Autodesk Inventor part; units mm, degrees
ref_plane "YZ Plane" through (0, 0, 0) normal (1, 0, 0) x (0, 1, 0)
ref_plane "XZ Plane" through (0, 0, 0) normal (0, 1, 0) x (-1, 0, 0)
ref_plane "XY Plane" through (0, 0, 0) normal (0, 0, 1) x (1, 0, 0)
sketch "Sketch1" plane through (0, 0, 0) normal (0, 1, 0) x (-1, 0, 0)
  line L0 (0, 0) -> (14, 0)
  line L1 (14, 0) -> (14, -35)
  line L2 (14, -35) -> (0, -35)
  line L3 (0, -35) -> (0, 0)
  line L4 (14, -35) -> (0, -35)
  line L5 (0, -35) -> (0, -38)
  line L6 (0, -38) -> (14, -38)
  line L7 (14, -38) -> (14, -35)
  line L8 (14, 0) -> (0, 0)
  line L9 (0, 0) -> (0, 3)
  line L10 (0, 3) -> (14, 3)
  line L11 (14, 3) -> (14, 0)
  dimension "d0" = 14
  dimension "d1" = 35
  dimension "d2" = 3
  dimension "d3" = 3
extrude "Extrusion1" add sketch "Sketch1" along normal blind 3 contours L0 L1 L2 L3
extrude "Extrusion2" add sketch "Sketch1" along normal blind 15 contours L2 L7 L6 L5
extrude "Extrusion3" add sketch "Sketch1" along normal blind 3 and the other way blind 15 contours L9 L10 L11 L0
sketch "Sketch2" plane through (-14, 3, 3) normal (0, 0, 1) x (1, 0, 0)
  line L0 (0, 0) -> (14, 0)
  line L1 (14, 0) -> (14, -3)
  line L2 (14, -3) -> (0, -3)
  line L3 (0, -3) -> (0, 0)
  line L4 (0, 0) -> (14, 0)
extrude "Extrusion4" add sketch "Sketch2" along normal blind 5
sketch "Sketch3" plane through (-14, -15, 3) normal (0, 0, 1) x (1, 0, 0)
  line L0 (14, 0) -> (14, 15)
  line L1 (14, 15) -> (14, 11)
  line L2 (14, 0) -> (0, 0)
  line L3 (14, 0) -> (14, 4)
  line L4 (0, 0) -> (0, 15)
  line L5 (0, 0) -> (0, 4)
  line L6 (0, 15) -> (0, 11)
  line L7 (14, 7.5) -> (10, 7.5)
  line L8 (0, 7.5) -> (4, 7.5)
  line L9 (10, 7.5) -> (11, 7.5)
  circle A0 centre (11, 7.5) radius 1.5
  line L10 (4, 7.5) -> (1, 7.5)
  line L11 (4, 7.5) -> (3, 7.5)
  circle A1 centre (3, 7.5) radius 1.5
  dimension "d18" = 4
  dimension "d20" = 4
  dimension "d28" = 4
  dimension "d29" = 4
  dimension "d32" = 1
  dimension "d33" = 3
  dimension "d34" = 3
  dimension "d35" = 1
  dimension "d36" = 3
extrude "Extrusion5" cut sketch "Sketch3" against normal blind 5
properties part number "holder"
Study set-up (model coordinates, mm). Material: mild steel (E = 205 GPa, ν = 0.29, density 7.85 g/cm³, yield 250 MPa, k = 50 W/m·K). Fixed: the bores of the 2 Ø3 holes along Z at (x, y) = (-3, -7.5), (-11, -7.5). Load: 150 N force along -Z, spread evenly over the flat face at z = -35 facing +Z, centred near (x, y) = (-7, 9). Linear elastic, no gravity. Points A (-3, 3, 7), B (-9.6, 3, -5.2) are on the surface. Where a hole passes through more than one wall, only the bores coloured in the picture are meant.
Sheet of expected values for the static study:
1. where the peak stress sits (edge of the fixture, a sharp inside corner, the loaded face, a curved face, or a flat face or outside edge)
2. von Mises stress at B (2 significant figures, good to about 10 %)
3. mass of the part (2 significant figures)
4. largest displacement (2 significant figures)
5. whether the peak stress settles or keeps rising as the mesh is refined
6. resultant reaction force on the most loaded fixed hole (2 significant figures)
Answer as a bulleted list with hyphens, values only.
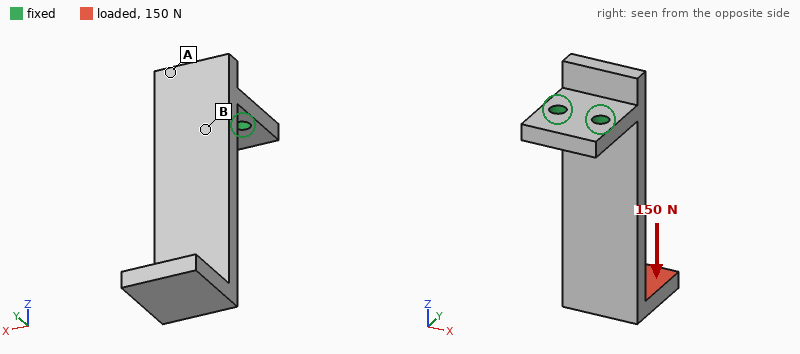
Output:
- edge of the fixture
- 55 MPa
- 24 g
- 0.25 mm
- keeps rising
- 76 N
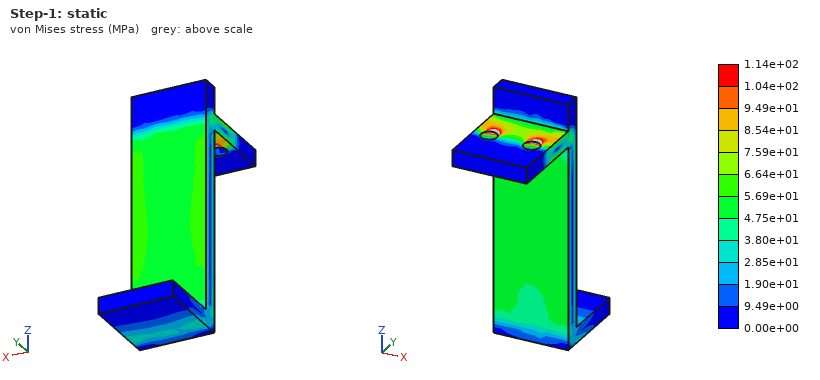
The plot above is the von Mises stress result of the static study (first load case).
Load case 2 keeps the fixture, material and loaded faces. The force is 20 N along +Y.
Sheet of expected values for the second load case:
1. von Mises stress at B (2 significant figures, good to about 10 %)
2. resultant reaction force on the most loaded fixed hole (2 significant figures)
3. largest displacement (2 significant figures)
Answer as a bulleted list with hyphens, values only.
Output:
- 27 MPa
- 12 N
- 95 µm
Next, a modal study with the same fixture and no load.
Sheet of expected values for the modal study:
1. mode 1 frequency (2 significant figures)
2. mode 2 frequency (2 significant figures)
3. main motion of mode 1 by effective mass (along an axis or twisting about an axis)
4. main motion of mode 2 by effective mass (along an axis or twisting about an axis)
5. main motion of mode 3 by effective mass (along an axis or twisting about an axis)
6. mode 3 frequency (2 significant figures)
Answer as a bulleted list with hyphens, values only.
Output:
- 840 Hz
- 2000 Hz
- along Y
- along X
- twisting about Z
- 4600 Hz
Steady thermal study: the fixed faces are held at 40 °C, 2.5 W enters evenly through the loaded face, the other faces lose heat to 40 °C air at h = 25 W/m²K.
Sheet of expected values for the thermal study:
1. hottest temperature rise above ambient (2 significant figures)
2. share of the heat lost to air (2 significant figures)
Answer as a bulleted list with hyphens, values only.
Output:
- 43 K
- 41 %
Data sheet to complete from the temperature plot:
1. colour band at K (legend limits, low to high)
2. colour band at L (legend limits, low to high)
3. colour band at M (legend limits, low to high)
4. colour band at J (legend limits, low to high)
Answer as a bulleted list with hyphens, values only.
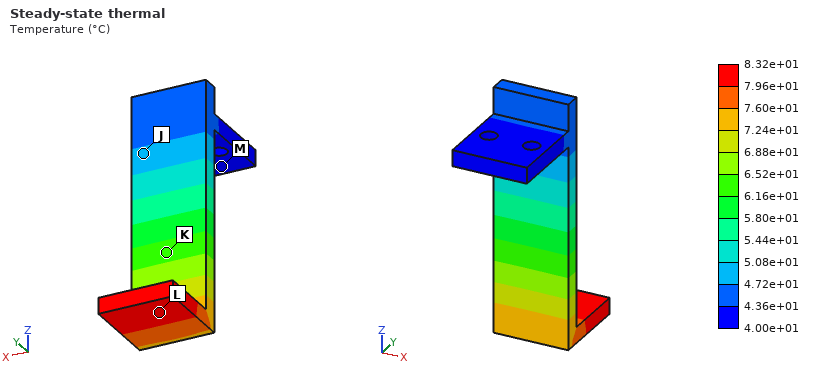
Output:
- 6.16e+01 to 6.52e+01 °C
- 7.96e+01 to 8.32e+01 °C
- 4.00e+01 to 4.36e+01 °C
- 4.72e+01 to 5.08e+01 °C
